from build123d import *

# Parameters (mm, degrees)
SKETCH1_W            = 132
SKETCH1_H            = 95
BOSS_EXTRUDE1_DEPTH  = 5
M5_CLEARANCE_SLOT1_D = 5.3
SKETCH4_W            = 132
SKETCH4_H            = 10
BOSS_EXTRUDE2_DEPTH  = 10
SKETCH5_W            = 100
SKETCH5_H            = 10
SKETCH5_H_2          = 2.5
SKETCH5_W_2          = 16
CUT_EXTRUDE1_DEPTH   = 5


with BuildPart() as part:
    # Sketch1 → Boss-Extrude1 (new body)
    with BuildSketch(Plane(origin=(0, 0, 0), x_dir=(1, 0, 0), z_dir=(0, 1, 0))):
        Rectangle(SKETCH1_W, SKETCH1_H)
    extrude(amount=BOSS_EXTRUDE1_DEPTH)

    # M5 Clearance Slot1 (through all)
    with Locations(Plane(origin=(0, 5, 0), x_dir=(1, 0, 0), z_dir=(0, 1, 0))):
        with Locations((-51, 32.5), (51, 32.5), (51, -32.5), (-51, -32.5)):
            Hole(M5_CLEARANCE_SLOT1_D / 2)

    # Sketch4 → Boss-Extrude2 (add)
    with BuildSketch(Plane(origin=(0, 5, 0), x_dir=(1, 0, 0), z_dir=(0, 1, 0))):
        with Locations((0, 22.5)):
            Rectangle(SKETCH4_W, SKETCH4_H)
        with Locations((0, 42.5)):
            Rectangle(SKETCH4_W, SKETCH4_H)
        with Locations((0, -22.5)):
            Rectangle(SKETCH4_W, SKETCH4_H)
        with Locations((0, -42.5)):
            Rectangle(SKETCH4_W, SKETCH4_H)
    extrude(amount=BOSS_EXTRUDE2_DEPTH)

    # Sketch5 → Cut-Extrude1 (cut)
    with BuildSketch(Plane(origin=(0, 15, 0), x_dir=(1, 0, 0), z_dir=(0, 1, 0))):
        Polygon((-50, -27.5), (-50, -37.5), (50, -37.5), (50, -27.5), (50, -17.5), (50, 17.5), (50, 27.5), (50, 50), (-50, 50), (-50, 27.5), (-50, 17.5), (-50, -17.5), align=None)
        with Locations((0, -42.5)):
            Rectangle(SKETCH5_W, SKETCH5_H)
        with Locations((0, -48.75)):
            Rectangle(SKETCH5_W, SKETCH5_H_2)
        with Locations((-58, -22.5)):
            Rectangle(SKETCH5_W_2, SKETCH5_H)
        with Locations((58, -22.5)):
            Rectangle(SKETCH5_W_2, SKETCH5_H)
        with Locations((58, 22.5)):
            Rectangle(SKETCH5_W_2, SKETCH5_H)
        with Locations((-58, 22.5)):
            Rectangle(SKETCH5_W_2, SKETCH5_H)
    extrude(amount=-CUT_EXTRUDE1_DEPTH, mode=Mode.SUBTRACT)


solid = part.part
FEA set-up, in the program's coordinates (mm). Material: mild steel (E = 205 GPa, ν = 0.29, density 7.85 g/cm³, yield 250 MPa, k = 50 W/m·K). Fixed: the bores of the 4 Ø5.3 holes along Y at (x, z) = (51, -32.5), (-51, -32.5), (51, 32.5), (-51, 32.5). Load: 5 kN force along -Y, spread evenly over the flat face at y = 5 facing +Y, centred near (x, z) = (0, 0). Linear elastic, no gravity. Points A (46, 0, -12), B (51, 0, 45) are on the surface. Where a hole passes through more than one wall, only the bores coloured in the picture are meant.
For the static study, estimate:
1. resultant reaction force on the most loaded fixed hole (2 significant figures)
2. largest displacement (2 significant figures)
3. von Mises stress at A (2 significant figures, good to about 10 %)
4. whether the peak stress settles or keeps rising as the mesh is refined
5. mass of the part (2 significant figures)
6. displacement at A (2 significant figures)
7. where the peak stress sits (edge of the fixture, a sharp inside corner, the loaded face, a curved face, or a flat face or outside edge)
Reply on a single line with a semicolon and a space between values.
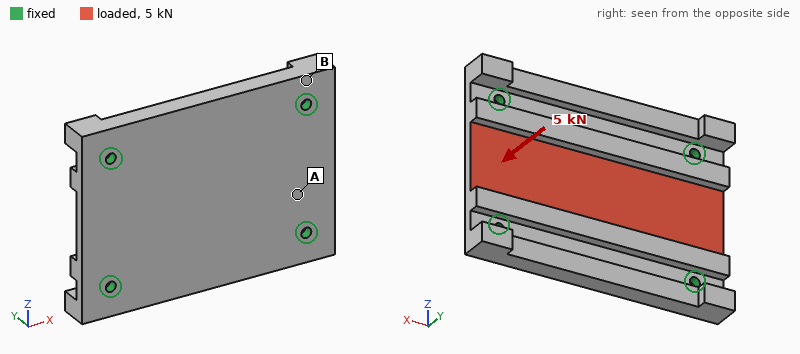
1.4 kN; 56 µm; 30 MPa; keeps rising; 720 g; 25 µm; edge of the fixture
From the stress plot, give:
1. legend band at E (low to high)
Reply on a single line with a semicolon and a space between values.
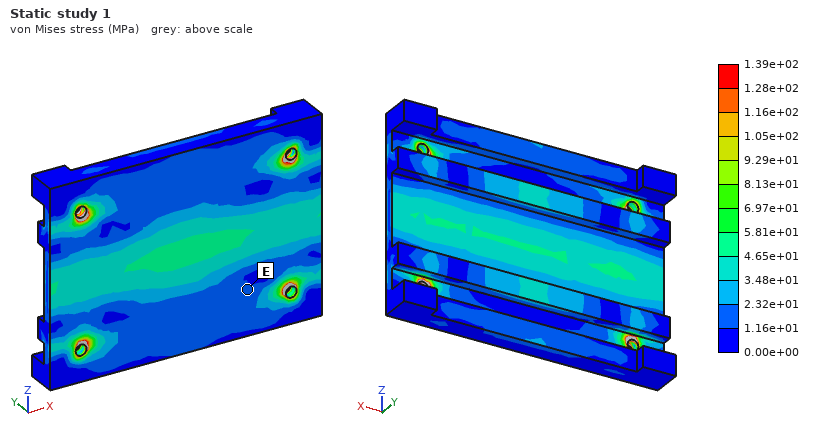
1.16e+01 to 2.32e+01 MPa
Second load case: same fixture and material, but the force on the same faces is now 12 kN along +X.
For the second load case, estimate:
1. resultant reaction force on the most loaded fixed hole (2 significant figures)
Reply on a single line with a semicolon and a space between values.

3.1 kN
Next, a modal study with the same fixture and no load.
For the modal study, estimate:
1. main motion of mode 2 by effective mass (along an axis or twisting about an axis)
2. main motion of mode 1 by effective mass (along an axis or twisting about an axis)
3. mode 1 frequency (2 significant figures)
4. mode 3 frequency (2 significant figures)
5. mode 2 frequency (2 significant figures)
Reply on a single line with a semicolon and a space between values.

twisting about X; along Y; 2900 Hz; 4500 Hz; 3800 Hz
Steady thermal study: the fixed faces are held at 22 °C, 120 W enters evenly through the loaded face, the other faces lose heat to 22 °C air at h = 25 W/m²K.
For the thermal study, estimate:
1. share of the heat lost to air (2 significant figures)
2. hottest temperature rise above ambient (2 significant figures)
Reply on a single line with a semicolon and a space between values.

20 %; 68 K
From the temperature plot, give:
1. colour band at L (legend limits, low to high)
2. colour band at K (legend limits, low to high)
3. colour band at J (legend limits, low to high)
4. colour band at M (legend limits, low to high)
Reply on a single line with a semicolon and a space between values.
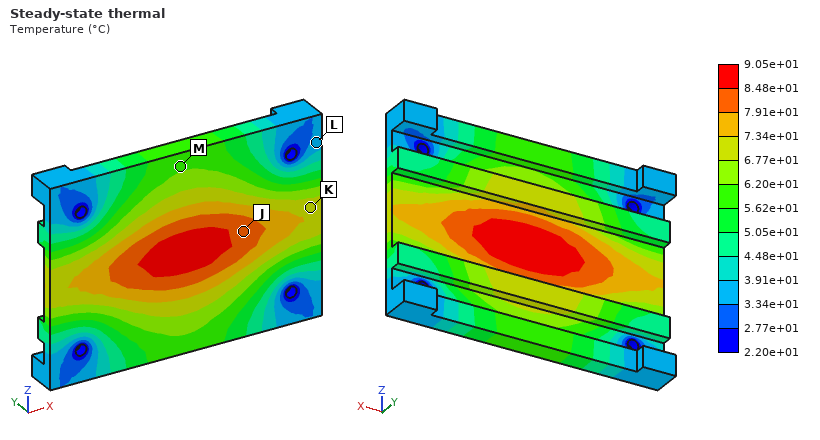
3.34e+01 to 3.91e+01 °C; 6.77e+01 to 7.34e+01 °C; 7.91e+01 to 8.48e+01 °C; 5.62e+01 to 6.20e+01 °C
